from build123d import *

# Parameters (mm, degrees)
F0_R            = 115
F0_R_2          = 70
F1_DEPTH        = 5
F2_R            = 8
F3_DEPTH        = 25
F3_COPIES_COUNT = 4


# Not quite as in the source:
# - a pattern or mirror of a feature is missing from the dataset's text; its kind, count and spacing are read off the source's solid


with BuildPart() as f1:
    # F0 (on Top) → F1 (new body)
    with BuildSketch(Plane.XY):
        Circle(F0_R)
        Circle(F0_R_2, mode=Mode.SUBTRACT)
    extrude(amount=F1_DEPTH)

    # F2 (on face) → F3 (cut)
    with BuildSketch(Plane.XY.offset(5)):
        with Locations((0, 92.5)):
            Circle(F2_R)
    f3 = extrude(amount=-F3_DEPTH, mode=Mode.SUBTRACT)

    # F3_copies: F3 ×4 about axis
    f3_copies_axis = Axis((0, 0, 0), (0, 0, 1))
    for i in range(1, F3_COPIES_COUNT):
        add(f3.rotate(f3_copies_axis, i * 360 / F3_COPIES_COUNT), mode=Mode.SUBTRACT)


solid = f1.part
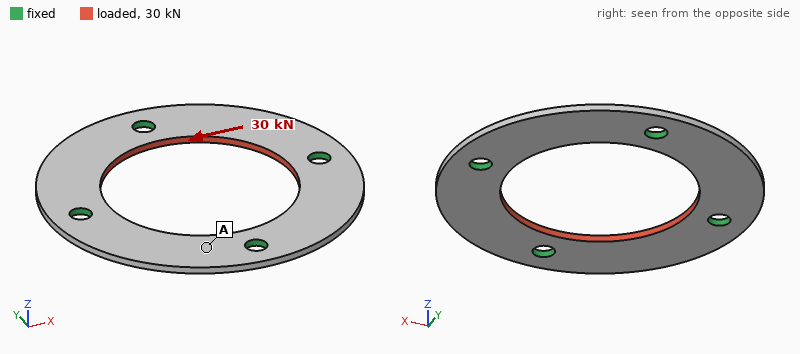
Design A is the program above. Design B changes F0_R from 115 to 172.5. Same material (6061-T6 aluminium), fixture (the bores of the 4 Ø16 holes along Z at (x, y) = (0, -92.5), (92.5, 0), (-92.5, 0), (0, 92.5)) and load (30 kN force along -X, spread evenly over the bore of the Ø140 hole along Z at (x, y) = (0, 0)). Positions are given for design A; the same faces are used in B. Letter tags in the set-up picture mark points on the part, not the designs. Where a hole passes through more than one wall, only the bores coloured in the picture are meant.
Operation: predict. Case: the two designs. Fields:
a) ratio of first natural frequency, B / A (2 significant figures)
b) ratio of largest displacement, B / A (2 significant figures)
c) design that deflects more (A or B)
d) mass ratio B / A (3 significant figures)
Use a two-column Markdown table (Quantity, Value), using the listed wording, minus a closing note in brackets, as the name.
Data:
| Quantity | Value |
|---|---|
| ratio of first natural frequency, B / A | 0.31 |
| ratio of largest displacement, B / A | 0.64 |
| design that deflects more | A |
| mass ratio B / A | 3.05 |
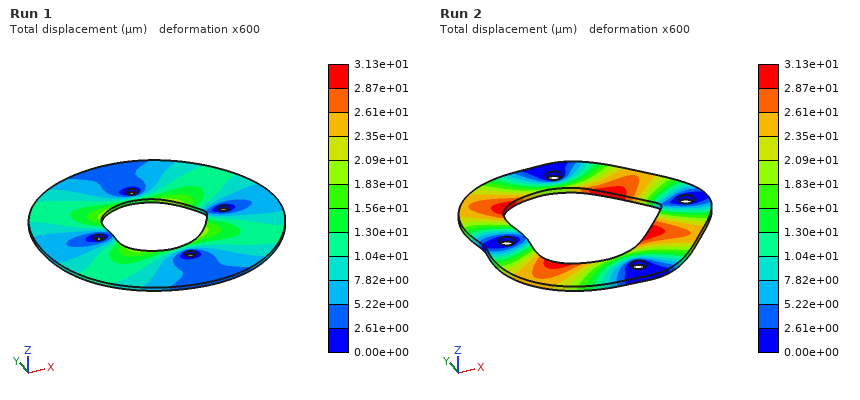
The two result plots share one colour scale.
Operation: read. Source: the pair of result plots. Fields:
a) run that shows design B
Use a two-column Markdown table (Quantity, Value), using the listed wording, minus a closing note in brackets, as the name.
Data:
| Quantity | Value |
|---|---|
| run that shows design B | Run 1 |
